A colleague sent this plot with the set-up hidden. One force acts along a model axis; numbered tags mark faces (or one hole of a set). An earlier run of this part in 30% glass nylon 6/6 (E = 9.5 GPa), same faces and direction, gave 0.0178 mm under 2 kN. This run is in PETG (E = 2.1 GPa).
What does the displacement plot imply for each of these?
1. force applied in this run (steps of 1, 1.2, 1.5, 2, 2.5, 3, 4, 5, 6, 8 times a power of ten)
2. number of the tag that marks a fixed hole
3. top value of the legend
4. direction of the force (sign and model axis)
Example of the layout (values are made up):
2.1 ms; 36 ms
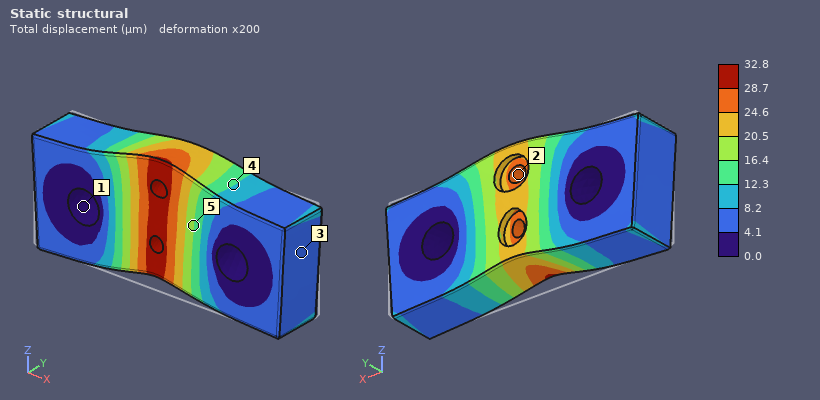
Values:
800 N; 1; 32.8 µm; +Z
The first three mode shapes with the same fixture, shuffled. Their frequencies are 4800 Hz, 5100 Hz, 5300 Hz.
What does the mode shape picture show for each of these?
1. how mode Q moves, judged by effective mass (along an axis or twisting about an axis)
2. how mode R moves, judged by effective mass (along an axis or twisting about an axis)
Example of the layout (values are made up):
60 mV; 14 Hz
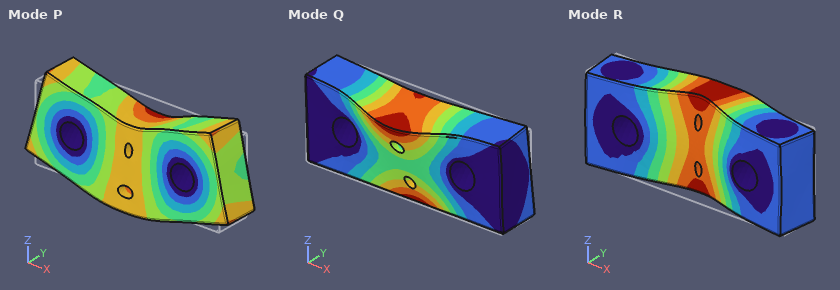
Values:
twisting about X; along Y
